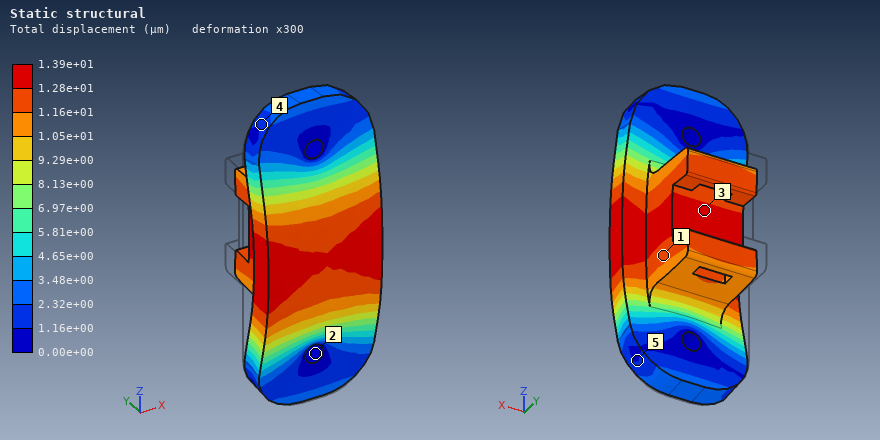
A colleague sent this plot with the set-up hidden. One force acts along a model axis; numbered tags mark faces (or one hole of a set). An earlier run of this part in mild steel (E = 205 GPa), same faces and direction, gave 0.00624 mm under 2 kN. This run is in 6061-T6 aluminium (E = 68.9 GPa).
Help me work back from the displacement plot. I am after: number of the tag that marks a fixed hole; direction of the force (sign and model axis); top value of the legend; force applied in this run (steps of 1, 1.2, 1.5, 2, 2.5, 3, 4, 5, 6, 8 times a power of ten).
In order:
2
-Y
1.39e+01 µm
1.5 kN
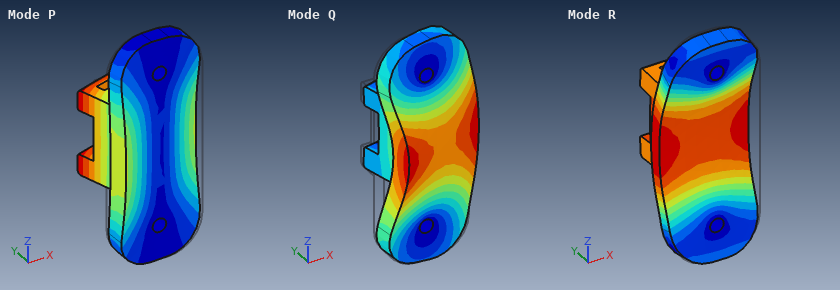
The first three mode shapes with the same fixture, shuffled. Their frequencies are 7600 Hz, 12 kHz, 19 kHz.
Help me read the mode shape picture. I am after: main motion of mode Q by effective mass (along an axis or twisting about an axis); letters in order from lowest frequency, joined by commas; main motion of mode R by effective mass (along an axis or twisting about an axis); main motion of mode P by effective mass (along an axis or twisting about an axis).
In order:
along X
P, R, Q
along Y
along X
